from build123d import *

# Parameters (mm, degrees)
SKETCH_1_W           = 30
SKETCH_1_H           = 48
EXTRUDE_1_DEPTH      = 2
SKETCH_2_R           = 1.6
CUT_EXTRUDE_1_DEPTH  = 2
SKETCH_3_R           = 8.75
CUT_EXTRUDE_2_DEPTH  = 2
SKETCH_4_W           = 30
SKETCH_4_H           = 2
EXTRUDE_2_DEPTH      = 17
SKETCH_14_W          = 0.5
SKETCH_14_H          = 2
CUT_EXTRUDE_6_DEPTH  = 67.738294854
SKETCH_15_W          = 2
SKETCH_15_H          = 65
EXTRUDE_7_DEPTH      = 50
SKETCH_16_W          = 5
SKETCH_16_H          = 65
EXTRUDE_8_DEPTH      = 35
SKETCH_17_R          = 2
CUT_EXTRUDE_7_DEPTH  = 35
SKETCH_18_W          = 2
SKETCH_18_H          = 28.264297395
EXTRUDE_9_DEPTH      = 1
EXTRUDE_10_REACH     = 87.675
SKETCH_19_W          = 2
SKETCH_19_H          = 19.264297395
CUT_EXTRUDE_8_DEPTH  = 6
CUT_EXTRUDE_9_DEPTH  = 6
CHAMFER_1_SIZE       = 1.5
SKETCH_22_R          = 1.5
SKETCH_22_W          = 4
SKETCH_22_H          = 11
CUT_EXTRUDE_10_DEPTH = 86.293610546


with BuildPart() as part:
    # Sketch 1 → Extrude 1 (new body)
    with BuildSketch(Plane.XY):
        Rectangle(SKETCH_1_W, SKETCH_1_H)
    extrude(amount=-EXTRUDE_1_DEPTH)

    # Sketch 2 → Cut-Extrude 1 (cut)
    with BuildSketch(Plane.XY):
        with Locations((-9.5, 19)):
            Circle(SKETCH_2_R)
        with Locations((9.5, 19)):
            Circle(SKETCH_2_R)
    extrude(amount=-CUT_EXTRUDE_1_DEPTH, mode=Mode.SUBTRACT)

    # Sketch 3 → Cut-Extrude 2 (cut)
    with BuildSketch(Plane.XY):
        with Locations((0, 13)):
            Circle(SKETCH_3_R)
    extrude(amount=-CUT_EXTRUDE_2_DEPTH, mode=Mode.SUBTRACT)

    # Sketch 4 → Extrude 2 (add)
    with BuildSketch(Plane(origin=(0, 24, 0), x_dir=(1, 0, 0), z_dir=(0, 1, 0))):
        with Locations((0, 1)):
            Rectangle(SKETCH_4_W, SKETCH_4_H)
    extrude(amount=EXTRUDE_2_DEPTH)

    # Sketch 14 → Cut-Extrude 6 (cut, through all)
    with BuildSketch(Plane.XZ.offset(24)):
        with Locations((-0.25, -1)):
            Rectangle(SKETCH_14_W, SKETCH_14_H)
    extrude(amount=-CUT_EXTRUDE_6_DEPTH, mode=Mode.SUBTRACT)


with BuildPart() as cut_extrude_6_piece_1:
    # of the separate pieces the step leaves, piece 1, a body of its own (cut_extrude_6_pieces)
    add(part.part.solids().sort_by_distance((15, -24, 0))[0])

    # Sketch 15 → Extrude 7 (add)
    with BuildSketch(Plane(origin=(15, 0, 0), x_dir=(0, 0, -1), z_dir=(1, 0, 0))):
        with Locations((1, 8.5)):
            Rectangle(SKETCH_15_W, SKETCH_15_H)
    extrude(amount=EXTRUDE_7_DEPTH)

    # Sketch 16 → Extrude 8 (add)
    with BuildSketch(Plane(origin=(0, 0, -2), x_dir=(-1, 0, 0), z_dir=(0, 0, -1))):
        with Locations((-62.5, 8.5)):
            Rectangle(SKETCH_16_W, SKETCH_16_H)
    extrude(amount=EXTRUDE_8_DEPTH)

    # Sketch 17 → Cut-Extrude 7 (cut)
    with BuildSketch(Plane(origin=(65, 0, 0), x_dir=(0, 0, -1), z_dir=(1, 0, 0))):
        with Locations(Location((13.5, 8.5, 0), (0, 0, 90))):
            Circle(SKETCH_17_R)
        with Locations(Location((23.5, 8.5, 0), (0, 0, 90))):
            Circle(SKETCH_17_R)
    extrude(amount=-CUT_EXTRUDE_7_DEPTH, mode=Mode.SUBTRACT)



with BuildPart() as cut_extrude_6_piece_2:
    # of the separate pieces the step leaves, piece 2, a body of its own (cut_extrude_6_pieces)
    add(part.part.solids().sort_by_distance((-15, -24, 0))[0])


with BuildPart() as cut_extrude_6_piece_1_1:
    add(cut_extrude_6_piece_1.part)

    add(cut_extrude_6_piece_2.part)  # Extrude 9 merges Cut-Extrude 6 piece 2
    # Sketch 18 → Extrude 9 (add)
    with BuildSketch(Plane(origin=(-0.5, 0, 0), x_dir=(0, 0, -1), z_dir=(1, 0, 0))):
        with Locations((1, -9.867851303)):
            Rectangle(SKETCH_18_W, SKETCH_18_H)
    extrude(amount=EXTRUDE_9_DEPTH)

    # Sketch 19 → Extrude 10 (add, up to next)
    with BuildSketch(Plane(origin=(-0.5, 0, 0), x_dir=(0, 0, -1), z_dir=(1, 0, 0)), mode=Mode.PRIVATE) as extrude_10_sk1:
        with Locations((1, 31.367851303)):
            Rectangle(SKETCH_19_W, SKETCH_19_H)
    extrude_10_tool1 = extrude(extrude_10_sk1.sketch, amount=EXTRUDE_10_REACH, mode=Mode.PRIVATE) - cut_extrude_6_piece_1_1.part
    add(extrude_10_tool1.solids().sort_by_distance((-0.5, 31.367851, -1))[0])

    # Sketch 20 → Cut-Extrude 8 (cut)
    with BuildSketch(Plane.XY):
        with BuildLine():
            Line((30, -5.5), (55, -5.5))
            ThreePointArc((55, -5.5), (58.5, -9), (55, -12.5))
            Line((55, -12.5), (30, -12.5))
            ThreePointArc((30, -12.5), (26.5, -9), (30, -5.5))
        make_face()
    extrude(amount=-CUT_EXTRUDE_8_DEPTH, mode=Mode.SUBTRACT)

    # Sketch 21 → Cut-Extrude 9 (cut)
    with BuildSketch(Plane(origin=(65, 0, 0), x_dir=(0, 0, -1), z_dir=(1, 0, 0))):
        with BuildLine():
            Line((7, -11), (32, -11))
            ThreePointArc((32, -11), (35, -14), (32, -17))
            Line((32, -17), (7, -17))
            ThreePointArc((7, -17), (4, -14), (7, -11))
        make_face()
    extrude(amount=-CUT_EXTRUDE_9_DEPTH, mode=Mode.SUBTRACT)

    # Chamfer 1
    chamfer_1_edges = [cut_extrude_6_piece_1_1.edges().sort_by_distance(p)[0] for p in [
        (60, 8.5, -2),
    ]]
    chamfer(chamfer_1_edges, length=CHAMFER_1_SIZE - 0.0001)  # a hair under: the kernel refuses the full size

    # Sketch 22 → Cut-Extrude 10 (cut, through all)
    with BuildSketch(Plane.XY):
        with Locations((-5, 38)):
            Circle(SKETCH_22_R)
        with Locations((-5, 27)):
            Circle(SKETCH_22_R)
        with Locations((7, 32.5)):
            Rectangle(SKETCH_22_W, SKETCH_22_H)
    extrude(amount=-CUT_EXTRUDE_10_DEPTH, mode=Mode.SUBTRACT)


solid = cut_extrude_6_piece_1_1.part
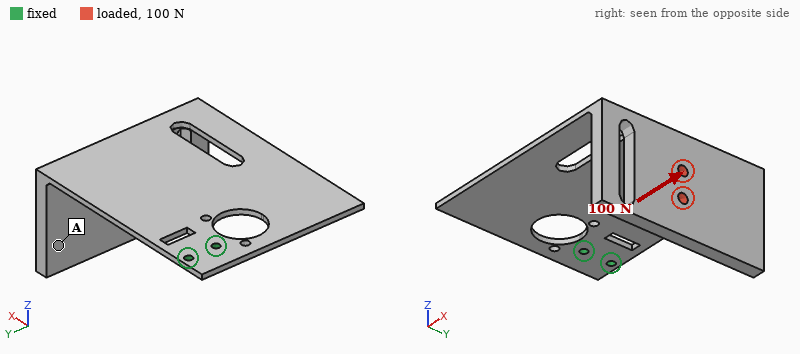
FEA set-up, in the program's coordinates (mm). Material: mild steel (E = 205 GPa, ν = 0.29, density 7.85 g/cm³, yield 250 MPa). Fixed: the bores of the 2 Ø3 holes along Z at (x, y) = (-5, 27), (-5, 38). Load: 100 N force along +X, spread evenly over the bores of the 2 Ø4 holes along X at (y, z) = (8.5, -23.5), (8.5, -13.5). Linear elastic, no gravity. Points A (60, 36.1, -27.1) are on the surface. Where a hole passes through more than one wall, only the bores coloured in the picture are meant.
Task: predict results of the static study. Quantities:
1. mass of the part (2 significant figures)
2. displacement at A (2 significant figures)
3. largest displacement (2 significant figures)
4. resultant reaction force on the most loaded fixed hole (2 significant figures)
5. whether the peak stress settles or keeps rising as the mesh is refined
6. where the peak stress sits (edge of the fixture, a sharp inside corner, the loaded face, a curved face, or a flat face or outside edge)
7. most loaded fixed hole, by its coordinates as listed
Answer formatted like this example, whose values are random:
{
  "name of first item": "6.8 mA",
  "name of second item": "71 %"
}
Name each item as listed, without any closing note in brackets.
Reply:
{
  "mass of the part": "160 g",
  "displacement at A": "0.96 mm",
  "largest displacement": "1.3 mm",
  "resultant reaction force on the most loaded fixed hole": "230 N",
  "whether the peak stress settles or keeps rising as the mesh is refined": "keeps rising",
  "where the peak stress sits": "edge of the fixture",
  "most loaded fixed hole, by its coordinates as listed": "(-5, 27)"
}
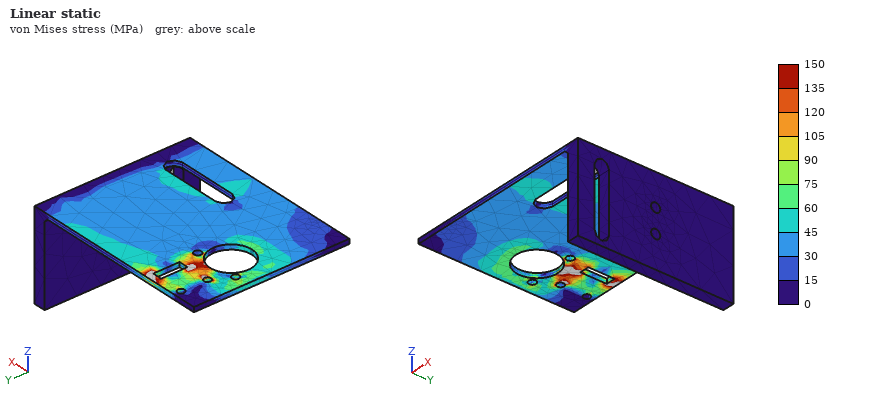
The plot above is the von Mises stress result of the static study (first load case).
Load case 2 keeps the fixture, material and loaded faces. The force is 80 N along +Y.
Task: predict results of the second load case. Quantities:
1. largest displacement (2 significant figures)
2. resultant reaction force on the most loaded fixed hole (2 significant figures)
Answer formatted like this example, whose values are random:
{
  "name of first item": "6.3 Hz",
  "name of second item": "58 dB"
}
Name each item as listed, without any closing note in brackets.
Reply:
{
  "largest displacement": "0.64 mm",
  "resultant reaction force on the most loaded fixed hole": "420 N"
}
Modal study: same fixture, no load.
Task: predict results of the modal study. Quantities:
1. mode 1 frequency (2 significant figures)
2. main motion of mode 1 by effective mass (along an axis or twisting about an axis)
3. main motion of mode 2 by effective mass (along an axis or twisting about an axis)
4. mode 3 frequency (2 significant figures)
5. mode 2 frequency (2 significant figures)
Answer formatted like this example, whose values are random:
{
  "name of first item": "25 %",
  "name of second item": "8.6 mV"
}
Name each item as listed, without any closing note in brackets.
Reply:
{
  "mode 1 frequency": "87 Hz",
  "main motion of mode 1 by effective mass": "along Z",
  "main motion of mode 2 by effective mass": "along Y",
  "mode 3 frequency": "530 Hz",
  "mode 2 frequency": "210 Hz"
}
